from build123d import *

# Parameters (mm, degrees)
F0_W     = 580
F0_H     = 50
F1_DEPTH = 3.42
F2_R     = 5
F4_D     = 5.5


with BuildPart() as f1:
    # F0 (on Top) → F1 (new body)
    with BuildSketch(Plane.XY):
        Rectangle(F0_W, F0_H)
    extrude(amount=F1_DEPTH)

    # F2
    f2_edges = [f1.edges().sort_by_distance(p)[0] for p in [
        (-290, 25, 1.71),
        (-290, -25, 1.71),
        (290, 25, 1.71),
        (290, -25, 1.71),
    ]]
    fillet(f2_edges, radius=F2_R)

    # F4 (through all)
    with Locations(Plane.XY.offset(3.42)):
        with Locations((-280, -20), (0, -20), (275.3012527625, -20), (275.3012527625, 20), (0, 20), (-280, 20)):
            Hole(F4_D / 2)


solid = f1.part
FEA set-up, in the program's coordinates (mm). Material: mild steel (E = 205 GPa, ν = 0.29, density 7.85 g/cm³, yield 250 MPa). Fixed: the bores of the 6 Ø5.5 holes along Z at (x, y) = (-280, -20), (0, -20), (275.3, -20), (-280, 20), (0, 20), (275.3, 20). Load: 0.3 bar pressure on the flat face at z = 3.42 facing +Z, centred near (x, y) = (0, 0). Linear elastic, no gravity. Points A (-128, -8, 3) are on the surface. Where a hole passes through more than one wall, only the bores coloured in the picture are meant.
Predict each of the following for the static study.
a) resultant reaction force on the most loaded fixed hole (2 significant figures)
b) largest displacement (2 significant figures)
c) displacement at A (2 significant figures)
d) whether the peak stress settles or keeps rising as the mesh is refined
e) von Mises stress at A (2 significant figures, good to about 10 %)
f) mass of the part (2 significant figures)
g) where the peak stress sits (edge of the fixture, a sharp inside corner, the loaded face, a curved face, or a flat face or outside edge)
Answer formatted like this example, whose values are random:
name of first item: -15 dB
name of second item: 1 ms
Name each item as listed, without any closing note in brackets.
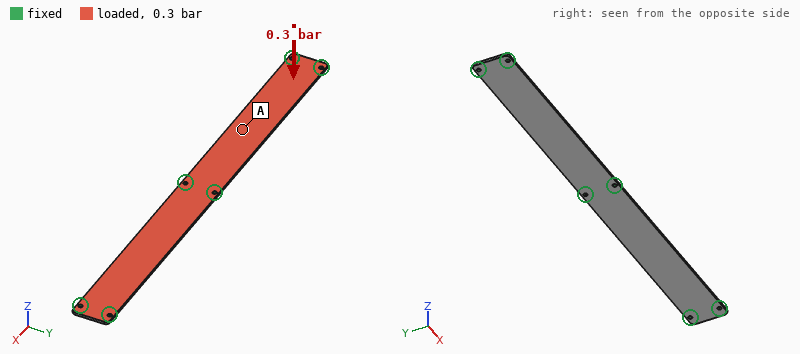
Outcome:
resultant reaction force on the most loaded fixed hole: 210 N
largest displacement: 0.70 mm
displacement at A: 0.67 mm
whether the peak stress settles or keeps rising as the mesh is refined: keeps rising
von Mises stress at A: 48 MPa
mass of the part: 770 g
where the peak stress sits: edge of the fixture
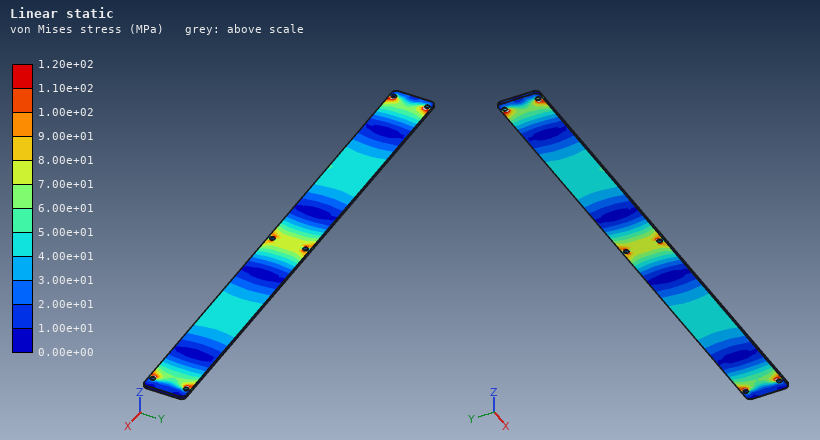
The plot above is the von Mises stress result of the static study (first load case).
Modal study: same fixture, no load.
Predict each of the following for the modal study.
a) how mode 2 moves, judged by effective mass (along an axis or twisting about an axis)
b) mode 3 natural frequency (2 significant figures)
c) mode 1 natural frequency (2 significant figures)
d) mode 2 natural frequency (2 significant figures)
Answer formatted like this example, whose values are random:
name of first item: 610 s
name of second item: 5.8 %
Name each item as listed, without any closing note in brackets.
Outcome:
how mode 2 moves, judged by effective mass: along Z
mode 3 natural frequency: 630 Hz
mode 1 natural frequency: 230 Hz
mode 2 natural frequency: 240 Hz
